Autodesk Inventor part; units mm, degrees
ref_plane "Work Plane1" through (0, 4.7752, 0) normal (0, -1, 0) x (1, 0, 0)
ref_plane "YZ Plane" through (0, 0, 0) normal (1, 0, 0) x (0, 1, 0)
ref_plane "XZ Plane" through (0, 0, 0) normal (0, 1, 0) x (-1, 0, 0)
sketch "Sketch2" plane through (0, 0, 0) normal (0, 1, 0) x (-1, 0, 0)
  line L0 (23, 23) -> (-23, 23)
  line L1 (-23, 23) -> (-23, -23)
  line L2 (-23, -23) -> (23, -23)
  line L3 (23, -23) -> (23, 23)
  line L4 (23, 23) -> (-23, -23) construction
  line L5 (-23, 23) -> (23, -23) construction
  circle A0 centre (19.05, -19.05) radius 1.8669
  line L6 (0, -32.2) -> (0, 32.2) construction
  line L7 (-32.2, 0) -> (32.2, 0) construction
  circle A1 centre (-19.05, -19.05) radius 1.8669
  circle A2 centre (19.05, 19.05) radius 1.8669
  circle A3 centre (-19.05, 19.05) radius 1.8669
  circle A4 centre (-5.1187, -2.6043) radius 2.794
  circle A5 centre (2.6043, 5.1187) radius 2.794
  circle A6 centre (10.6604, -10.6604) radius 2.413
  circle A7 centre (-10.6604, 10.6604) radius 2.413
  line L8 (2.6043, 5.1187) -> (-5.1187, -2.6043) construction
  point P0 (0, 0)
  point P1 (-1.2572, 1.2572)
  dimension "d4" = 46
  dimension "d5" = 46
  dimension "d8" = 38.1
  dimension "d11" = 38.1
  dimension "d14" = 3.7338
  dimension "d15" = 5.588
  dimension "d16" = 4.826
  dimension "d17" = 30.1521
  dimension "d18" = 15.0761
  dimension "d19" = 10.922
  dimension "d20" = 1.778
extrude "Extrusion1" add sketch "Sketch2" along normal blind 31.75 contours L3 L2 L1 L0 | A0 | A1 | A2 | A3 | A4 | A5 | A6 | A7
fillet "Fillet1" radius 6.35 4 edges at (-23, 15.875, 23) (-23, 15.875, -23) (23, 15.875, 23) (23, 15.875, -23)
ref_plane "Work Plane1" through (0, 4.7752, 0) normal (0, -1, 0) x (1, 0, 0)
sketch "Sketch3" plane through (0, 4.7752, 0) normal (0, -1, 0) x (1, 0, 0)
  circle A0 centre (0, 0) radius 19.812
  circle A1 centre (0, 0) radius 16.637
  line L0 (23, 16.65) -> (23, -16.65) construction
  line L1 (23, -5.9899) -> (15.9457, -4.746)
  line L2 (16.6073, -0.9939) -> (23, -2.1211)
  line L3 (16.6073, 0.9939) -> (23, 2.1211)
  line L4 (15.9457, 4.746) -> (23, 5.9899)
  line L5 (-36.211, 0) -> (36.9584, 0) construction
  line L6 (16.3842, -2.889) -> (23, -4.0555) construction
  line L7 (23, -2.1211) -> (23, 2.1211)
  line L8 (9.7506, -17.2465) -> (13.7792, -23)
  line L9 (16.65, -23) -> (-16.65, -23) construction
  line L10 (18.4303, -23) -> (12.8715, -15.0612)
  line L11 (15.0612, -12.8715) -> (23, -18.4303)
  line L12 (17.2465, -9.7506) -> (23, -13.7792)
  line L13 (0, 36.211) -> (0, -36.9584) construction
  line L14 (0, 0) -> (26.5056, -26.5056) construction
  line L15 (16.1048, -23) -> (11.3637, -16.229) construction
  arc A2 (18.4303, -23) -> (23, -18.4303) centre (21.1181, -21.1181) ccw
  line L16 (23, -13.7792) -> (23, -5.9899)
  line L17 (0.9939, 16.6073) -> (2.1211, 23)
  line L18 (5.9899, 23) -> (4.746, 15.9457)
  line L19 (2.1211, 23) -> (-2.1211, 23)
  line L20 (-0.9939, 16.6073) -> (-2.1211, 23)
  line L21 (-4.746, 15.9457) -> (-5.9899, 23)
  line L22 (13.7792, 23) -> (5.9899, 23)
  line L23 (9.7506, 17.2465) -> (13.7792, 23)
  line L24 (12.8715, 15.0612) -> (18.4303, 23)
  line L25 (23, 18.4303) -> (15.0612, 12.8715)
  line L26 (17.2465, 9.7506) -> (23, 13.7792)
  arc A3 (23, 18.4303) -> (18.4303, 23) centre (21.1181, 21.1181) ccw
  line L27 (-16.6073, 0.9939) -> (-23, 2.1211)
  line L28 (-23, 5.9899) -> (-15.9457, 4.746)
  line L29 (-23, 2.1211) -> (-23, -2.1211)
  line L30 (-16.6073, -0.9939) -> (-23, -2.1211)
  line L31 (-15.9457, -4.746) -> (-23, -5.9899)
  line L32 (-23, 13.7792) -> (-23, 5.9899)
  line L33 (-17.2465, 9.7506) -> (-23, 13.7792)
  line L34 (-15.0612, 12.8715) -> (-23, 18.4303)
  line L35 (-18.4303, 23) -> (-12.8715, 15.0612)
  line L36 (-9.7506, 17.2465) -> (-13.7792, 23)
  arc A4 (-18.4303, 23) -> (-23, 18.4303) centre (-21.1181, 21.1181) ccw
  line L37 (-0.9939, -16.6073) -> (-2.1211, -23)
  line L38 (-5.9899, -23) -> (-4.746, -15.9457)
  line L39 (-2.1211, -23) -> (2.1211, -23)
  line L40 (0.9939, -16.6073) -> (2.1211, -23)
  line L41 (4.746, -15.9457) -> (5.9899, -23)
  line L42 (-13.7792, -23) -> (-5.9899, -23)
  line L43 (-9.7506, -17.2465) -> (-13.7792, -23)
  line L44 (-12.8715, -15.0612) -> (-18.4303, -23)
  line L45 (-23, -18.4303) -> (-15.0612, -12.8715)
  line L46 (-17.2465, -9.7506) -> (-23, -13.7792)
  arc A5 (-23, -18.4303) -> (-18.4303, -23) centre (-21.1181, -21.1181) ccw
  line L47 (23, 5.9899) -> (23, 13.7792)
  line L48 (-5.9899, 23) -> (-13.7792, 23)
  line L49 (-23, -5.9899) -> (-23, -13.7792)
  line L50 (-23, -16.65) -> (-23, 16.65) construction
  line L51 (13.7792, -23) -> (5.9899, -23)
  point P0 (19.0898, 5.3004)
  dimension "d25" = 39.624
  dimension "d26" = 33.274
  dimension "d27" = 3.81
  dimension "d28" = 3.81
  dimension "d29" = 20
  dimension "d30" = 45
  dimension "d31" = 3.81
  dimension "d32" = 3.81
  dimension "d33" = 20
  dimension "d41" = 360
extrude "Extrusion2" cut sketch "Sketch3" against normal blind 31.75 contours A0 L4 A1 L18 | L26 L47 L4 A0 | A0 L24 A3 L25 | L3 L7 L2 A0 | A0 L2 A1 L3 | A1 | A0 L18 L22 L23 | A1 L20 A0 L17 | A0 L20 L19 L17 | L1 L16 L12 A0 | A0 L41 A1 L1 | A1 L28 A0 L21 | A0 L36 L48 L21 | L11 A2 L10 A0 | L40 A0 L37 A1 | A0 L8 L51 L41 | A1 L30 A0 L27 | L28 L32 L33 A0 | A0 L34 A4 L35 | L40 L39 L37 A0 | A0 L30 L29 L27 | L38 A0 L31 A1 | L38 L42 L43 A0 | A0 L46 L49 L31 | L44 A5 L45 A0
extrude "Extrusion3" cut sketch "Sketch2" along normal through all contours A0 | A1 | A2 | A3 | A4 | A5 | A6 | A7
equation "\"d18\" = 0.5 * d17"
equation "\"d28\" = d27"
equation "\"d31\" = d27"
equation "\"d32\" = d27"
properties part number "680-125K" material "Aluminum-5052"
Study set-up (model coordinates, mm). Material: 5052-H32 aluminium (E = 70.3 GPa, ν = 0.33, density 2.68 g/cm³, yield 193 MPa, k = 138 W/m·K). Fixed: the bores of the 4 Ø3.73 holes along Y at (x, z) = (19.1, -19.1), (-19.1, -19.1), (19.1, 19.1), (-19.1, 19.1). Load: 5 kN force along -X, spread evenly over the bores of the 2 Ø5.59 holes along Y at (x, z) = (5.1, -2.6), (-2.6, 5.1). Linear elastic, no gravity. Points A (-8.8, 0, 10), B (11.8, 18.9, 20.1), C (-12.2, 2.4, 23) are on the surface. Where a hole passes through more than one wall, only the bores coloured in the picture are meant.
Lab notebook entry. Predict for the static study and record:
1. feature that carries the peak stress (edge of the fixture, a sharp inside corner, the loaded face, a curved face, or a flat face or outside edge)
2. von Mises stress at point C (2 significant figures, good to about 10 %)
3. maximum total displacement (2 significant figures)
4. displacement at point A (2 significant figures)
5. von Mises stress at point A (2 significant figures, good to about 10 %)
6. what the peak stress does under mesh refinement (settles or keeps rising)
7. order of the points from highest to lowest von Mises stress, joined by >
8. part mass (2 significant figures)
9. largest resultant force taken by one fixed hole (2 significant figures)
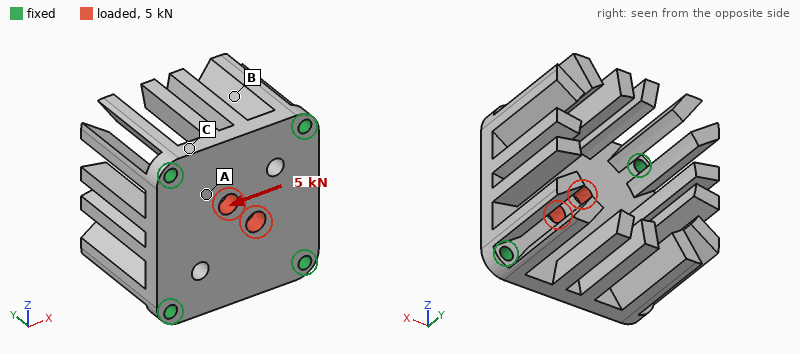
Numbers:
edge of the fixture
13 MPa
13 µm
6.7 µm
27 MPa
keeps rising
A > C > B
58 g
1.5 kN
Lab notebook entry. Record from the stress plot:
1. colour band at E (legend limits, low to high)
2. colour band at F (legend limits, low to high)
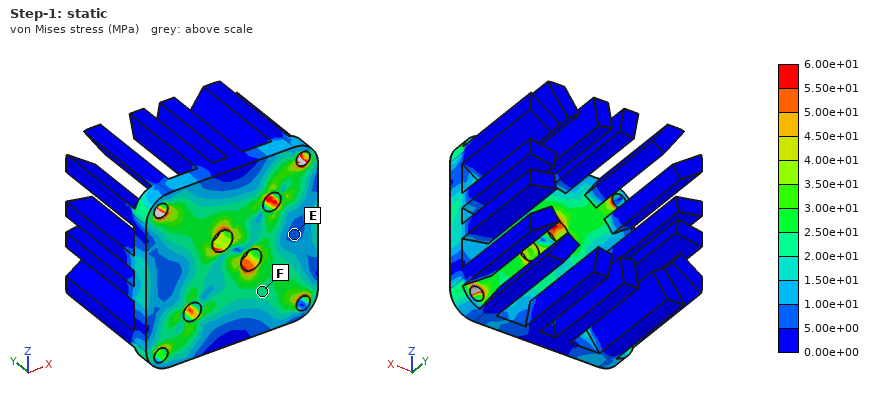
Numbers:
5.00e+00 to 1.00e+01 MPa
2.00e+01 to 2.50e+01 MPa
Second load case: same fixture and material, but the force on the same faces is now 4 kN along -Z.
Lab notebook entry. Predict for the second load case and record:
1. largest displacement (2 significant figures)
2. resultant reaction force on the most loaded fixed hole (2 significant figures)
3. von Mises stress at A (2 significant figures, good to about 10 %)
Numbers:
11 µm
1.2 kN
20 MPa
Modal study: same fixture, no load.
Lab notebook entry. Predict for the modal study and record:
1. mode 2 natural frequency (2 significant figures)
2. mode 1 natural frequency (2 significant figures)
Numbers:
3500 Hz
3400 Hz
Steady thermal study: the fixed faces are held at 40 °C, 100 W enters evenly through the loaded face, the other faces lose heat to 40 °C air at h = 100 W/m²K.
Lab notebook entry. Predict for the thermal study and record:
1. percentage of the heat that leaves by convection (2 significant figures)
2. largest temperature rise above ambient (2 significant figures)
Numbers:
20 %
56 K
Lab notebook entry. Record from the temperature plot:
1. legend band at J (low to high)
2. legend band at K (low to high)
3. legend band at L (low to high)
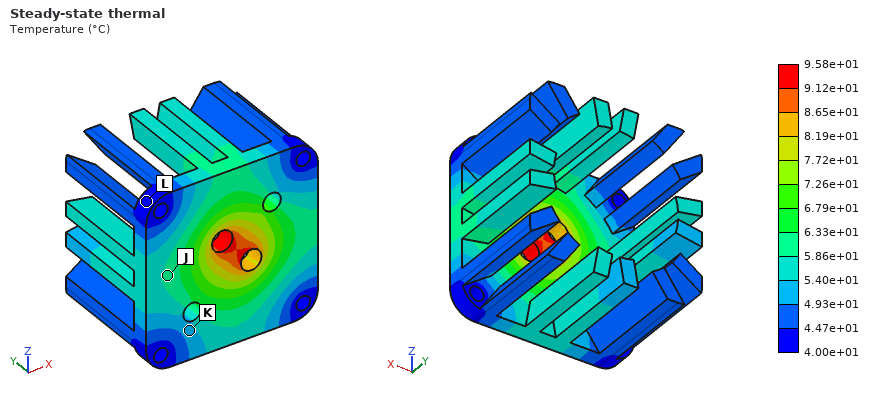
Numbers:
5.86e+01 to 6.33e+01 °C
4.93e+01 to 5.40e+01 °C
4.00e+01 to 4.47e+01 °C
